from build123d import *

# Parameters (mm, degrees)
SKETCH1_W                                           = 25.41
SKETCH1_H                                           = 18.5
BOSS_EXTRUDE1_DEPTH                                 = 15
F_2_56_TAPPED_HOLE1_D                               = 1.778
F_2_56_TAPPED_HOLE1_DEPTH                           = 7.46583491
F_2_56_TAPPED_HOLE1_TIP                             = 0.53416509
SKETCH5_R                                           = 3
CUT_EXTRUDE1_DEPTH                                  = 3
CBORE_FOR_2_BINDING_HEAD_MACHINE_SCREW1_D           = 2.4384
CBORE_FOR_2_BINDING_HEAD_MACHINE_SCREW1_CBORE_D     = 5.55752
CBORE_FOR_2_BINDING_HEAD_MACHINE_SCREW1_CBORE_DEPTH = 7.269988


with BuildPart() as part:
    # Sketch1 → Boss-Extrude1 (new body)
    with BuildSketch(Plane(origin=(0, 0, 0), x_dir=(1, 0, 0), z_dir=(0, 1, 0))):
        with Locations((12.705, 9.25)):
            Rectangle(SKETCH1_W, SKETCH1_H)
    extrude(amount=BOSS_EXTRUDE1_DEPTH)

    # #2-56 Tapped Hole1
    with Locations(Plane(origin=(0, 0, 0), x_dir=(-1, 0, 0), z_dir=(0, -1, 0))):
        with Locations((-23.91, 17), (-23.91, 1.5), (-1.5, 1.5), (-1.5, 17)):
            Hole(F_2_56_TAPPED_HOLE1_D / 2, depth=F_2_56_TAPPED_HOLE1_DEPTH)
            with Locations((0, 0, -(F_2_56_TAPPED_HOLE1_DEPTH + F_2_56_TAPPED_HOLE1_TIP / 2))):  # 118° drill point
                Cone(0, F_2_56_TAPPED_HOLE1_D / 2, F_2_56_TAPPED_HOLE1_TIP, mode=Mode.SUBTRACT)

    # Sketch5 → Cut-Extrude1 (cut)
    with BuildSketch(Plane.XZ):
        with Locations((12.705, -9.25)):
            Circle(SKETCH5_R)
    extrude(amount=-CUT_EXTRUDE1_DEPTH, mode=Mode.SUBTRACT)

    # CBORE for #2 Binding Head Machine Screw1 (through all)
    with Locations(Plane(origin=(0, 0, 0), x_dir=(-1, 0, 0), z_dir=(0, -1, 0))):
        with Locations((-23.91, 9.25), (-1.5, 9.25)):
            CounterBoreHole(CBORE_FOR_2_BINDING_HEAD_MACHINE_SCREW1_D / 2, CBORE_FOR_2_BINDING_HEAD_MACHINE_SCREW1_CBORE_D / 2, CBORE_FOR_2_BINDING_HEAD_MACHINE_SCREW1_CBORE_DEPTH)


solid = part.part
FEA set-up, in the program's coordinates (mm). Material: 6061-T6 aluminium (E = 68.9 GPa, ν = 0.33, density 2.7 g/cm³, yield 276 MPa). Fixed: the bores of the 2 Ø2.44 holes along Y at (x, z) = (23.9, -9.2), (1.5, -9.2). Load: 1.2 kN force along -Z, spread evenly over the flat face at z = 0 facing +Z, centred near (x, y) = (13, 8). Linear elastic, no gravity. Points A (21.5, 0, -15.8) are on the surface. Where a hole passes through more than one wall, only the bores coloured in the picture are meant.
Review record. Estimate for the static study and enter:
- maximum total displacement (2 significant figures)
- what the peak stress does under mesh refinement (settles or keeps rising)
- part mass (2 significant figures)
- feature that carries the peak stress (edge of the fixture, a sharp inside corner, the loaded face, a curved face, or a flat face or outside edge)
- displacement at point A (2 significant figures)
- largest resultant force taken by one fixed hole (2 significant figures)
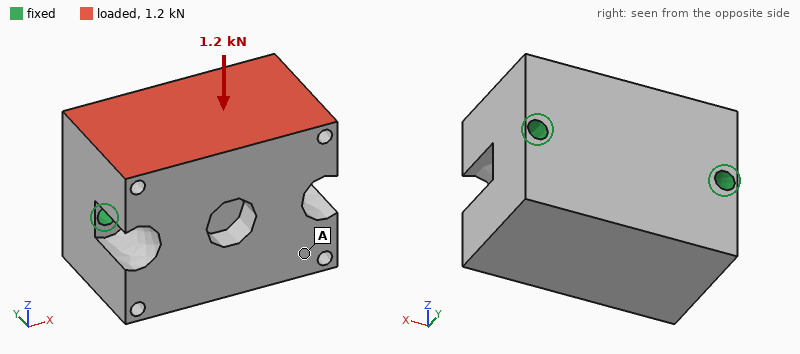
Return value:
6.2 µm
keeps rising
18 g
edge of the fixture
4.7 µm
600 N
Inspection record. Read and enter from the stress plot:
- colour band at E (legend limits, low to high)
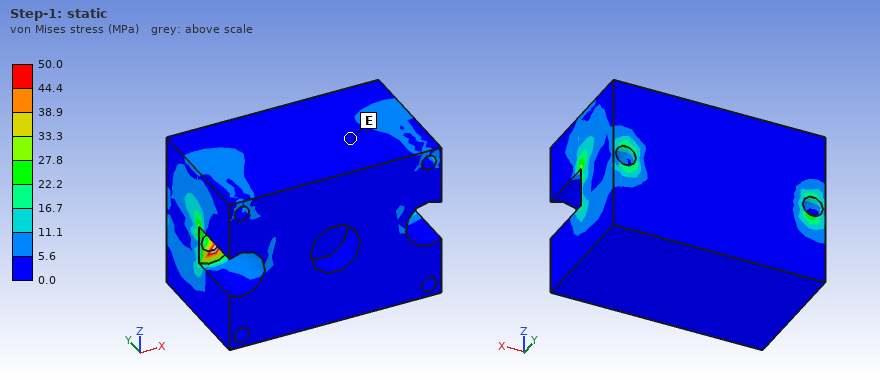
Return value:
0.0 to 5.6 MPa
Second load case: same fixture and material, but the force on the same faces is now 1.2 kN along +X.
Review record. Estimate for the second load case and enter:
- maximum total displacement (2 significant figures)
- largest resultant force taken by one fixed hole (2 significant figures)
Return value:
4.3 µm
790 N
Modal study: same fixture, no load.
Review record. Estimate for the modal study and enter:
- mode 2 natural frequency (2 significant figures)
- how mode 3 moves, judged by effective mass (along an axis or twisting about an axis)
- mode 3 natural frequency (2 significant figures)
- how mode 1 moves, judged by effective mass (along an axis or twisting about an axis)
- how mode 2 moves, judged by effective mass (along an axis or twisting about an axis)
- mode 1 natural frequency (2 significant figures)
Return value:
34 kHz
along X
38 kHz
along Z
along Y
18 kHz
